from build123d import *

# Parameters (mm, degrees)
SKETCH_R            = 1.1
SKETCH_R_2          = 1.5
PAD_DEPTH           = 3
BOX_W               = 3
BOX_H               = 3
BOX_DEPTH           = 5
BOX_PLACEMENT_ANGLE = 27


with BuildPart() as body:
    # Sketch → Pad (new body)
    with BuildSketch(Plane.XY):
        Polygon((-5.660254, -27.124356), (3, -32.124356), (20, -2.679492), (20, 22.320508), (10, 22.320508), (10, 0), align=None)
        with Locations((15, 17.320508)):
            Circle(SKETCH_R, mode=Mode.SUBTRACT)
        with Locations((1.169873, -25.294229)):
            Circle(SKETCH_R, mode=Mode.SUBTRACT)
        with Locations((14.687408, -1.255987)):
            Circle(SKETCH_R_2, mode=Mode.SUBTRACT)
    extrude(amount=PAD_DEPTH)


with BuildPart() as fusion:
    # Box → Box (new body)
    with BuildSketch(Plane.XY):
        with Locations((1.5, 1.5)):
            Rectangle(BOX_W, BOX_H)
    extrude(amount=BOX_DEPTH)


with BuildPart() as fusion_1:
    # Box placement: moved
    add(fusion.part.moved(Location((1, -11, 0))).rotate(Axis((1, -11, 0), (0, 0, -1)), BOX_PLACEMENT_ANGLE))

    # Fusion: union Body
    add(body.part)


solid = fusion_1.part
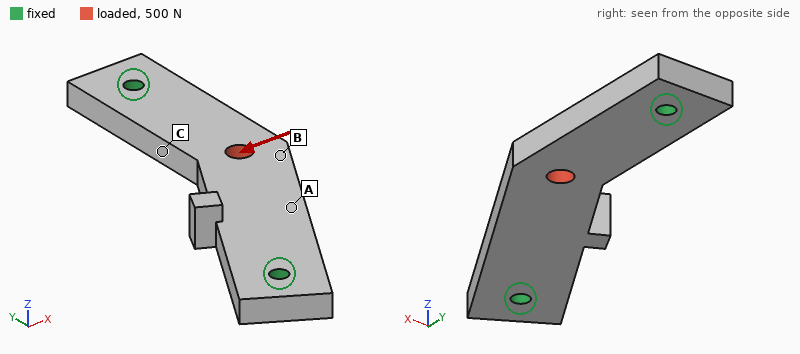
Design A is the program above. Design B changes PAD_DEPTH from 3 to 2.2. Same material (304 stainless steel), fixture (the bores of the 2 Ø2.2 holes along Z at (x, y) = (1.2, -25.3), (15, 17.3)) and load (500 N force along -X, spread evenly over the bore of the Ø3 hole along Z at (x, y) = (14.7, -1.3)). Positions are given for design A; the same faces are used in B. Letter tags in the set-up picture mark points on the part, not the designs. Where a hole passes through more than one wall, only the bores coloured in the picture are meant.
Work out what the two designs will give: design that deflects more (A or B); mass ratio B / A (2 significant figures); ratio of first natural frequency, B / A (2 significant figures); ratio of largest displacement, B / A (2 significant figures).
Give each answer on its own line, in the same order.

B
0.74
0.75
1.4
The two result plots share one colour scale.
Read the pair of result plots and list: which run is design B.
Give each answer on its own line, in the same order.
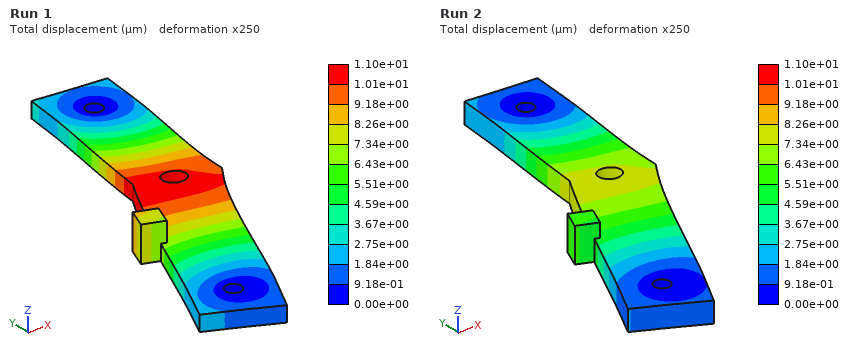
Run 1
